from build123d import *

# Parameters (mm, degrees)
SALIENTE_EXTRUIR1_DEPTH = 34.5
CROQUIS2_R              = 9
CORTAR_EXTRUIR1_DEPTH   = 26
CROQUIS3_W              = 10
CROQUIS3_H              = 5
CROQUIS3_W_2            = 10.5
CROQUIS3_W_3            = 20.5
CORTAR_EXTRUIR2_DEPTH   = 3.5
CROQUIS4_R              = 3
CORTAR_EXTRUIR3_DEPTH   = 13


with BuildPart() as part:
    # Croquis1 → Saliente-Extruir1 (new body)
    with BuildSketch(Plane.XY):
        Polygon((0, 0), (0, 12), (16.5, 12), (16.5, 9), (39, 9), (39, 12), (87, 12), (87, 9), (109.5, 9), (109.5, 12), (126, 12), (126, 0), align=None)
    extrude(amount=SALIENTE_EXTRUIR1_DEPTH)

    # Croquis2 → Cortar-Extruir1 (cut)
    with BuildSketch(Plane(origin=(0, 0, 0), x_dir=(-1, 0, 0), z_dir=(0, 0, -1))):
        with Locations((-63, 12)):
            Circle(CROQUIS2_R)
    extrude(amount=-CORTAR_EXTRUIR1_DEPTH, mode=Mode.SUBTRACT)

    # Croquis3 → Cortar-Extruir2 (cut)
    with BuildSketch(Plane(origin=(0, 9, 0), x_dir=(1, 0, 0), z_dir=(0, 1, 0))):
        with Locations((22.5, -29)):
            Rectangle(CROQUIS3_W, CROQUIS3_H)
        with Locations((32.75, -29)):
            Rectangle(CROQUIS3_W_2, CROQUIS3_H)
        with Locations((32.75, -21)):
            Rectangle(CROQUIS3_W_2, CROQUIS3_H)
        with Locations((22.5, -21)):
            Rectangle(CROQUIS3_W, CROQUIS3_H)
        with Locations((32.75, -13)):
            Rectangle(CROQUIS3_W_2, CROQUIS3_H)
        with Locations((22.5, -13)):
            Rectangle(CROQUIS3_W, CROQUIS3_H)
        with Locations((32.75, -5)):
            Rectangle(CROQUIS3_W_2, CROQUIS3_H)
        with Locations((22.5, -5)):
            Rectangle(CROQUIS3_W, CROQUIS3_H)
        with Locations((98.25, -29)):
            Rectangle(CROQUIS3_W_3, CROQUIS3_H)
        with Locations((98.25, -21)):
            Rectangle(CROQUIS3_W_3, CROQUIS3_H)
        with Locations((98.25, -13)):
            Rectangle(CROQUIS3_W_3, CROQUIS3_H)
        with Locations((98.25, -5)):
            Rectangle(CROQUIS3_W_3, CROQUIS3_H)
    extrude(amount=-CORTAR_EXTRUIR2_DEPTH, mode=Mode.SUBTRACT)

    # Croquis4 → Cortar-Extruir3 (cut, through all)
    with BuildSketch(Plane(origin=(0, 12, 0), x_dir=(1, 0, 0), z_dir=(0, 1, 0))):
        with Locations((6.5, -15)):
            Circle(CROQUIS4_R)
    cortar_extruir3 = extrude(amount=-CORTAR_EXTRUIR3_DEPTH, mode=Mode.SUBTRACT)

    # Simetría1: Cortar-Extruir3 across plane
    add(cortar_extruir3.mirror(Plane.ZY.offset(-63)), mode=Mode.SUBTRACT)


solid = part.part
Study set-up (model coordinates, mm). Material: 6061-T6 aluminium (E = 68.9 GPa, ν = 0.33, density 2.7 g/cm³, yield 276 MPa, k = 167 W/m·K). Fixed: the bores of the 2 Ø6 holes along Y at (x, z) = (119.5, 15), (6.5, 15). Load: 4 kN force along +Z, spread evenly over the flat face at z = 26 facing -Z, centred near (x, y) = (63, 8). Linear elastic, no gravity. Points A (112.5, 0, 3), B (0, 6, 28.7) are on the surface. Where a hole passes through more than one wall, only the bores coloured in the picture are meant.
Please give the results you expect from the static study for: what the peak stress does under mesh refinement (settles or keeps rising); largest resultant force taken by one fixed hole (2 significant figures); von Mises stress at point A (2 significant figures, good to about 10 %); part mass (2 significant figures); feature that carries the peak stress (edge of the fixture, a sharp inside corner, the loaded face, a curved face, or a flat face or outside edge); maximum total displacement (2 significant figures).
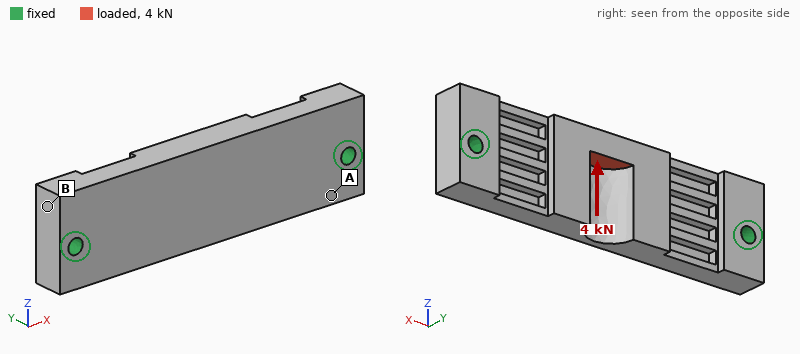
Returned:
keeps rising
2.5 kN
27 MPa
110 g
edge of the fixture
0.13 mm
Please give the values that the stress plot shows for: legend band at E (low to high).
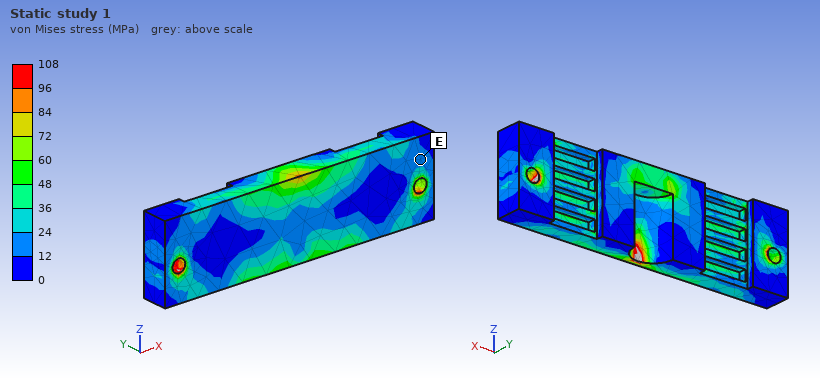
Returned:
12 to 24 MPa
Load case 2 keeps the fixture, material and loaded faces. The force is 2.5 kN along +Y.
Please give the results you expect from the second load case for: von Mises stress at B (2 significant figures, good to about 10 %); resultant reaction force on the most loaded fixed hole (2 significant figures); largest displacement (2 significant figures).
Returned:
16 MPa
1.5 kN
0.20 mm
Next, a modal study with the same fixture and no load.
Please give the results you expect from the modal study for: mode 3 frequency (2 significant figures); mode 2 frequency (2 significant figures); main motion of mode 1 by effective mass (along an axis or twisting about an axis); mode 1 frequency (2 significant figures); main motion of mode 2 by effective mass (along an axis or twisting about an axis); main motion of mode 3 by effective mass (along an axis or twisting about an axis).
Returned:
6500 Hz
5300 Hz
along Y
3400 Hz
along Z
along Z
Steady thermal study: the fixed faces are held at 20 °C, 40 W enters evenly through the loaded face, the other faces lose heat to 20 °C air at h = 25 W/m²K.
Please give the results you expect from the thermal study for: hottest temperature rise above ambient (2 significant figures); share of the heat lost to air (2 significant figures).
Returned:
34 K
8.9 %
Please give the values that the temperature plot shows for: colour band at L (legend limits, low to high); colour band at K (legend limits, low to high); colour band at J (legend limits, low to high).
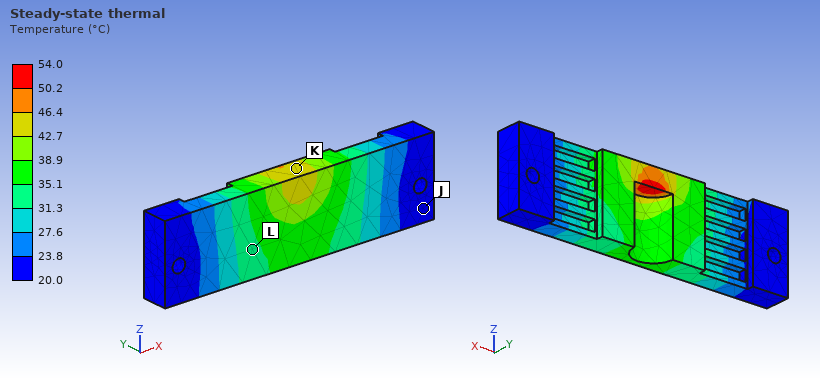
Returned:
31.3 to 35.1 °C
42.7 to 46.4 °C
20.0 to 23.8 °C
